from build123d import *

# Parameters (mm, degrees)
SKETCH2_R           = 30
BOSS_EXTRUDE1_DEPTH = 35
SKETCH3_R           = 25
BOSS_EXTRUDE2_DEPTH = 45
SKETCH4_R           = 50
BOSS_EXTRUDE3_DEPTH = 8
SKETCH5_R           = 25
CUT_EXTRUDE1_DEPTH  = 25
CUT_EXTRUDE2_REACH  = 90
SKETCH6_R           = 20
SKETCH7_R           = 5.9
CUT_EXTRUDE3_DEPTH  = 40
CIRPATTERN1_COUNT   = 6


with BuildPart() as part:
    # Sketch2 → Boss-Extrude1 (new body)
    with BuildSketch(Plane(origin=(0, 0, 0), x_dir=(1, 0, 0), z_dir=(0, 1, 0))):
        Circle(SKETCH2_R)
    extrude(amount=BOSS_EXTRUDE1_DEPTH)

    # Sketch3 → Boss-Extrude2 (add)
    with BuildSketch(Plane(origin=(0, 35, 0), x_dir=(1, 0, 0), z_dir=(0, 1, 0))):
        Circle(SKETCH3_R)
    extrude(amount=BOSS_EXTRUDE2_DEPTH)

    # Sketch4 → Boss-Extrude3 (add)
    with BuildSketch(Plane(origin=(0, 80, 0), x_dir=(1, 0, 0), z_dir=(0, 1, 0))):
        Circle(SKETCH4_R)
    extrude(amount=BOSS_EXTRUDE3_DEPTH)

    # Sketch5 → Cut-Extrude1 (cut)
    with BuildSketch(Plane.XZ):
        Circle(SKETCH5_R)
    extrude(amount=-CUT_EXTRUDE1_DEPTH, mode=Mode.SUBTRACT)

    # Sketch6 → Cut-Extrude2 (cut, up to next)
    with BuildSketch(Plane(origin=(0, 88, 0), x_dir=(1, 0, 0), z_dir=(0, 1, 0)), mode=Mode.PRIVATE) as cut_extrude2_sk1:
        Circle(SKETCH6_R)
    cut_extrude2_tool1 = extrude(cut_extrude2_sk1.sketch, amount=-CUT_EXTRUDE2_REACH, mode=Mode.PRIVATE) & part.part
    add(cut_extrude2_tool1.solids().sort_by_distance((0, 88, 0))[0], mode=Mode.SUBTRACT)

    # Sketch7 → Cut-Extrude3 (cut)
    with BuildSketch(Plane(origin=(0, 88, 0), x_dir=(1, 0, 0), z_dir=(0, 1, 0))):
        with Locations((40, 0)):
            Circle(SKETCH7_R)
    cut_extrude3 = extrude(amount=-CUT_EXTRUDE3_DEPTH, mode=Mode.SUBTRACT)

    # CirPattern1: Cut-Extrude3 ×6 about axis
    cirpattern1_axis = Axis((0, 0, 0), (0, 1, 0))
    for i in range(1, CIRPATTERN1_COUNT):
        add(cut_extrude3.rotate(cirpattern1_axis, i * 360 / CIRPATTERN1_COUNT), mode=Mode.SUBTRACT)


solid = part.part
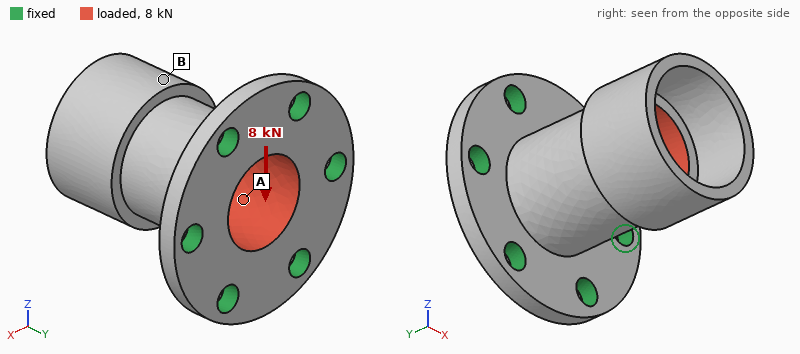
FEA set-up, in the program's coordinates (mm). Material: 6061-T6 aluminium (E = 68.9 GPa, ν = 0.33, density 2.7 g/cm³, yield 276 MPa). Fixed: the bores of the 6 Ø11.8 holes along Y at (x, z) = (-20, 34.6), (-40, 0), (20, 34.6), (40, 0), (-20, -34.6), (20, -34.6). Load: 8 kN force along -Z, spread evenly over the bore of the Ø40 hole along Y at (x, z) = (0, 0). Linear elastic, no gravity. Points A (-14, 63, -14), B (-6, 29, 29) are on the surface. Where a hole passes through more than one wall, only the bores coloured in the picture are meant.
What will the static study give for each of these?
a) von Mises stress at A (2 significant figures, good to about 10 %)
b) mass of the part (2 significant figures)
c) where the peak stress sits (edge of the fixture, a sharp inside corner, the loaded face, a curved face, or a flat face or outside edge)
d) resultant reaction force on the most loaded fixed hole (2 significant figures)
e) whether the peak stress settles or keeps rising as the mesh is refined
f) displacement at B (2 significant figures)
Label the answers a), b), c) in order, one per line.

a) 24 MPa
b) 310 g
c) edge of the fixture
d) 2.7 kN
e) keeps rising
f) 70 µm
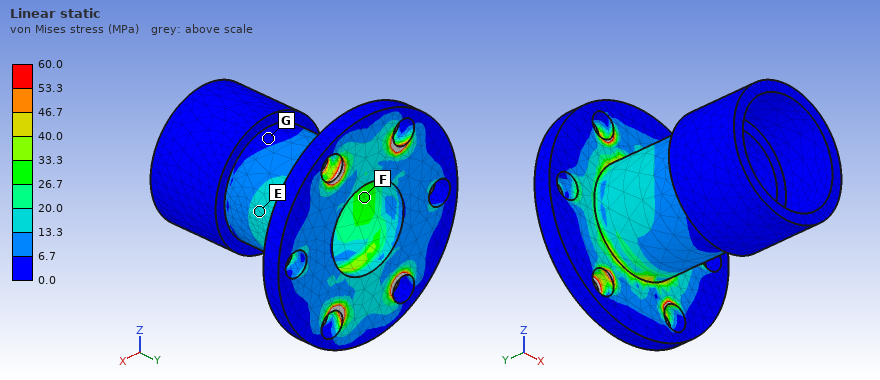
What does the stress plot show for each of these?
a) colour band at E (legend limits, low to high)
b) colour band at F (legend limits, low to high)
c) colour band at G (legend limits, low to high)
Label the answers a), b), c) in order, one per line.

a) 13.3 to 20.0 MPa
b) 26.7 to 33.3 MPa
c) 0.0 to 6.7 MPa
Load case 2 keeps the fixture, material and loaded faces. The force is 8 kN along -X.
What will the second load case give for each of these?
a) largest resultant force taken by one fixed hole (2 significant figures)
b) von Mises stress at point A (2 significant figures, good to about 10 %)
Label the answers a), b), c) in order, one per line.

a) 3.1 kN
b) 23 MPa
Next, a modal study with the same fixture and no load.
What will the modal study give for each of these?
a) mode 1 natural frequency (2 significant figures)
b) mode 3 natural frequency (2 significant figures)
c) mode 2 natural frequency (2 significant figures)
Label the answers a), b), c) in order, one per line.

a) 2900 Hz
b) 6100 Hz
c) 2900 Hz
